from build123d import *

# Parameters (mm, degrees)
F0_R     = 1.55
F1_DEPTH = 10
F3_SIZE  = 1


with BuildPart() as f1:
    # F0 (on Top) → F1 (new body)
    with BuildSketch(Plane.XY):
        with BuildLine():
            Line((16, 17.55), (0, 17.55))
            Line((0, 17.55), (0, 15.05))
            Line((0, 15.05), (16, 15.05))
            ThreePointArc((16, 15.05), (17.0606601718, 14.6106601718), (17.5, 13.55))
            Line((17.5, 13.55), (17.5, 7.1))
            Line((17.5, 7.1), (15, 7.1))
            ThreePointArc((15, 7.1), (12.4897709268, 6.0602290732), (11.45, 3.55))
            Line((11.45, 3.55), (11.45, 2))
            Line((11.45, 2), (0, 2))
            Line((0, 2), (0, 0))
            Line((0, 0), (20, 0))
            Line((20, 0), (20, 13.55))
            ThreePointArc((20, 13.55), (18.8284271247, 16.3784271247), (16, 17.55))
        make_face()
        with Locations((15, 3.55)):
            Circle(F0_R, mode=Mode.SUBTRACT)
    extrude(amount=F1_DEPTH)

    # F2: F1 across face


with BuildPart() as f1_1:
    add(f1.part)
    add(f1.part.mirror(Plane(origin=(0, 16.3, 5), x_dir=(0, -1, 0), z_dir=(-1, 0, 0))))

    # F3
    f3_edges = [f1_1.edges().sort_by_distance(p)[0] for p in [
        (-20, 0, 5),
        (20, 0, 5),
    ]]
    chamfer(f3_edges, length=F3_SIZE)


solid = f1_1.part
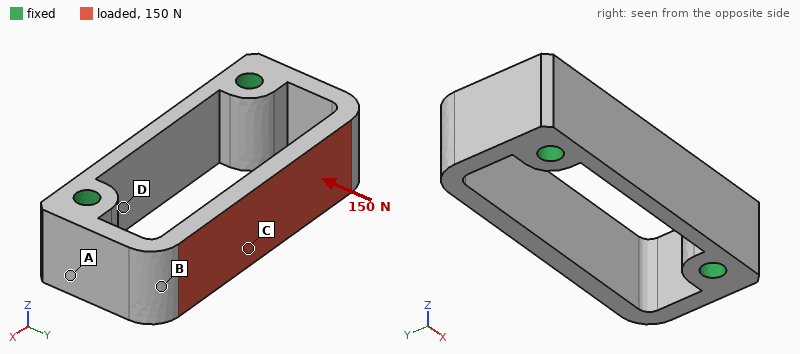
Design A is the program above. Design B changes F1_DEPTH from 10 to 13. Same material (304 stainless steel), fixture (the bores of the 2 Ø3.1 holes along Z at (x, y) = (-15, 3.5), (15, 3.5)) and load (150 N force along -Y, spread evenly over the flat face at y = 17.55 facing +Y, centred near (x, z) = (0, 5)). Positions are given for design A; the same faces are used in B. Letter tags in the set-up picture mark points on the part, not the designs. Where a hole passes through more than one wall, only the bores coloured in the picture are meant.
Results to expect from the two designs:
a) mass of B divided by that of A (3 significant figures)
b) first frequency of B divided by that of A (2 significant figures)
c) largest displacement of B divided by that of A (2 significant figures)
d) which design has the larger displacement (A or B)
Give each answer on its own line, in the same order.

1.30
1.0
0.77
A
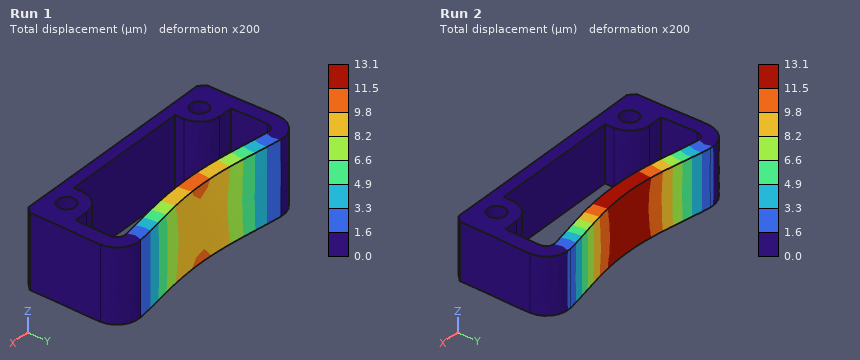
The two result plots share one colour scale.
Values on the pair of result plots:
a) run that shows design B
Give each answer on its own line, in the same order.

Run 1
